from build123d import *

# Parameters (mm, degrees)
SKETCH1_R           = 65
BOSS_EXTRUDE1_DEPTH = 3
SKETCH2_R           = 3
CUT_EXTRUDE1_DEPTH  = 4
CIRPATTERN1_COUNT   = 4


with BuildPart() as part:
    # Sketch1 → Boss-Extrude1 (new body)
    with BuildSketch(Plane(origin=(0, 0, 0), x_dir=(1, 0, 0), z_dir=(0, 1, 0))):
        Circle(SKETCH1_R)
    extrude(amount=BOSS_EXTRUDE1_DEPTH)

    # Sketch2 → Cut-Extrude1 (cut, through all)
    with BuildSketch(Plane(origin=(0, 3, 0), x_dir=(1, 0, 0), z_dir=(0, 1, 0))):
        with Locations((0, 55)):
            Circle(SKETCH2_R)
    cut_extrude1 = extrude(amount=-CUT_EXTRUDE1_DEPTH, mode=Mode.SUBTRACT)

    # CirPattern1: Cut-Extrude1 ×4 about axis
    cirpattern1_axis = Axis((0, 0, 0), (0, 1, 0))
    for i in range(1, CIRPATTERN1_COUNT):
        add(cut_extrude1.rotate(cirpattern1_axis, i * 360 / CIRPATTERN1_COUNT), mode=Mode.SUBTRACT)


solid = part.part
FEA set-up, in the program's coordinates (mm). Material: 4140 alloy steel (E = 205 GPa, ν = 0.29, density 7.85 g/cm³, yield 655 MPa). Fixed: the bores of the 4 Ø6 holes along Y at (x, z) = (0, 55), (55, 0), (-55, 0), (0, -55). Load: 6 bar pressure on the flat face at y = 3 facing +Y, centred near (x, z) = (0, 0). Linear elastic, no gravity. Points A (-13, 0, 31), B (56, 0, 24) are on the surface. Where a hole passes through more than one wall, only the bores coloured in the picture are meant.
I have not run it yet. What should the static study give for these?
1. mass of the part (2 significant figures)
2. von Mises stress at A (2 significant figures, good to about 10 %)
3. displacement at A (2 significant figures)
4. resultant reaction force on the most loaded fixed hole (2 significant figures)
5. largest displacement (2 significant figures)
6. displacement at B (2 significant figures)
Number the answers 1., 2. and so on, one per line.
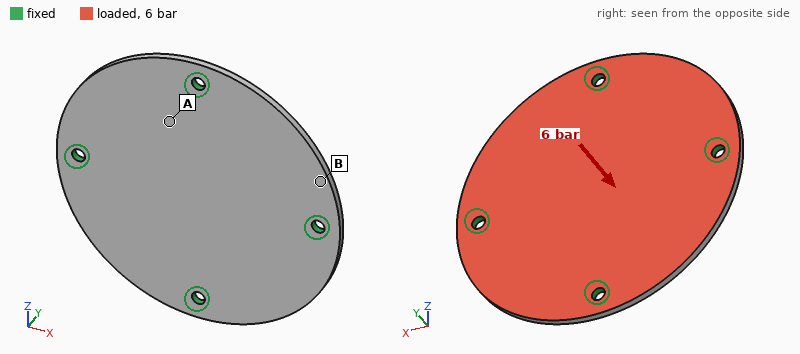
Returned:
1. 310 g
2. 100 MPa
3. 0.15 mm
4. 2.0 kN
5. 0.26 mm
6. 0.081 mm
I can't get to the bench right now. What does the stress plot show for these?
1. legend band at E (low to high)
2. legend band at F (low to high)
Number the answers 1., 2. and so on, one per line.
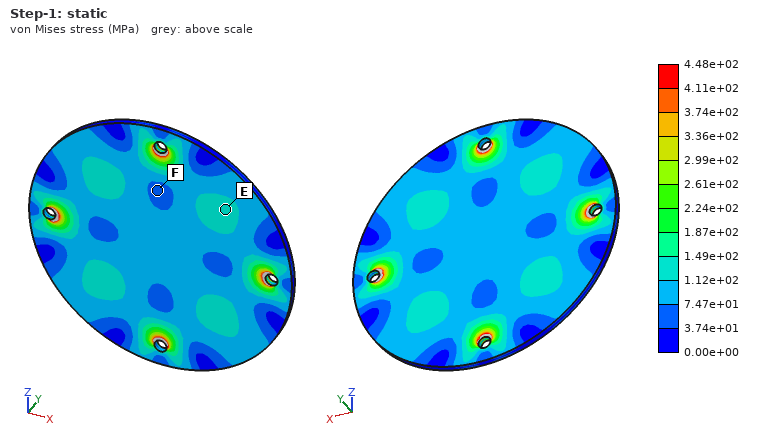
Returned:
1. 1.12e+02 to 1.49e+02 MPa
2. 3.74e+01 to 7.47e+01 MPa
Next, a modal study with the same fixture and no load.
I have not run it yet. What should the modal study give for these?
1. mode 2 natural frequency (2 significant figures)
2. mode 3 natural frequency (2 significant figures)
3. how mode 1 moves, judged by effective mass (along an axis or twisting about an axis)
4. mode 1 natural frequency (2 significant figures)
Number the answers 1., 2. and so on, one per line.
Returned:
1. 2100 Hz
2. 2200 Hz
3. along Y
4. 1900 Hz
